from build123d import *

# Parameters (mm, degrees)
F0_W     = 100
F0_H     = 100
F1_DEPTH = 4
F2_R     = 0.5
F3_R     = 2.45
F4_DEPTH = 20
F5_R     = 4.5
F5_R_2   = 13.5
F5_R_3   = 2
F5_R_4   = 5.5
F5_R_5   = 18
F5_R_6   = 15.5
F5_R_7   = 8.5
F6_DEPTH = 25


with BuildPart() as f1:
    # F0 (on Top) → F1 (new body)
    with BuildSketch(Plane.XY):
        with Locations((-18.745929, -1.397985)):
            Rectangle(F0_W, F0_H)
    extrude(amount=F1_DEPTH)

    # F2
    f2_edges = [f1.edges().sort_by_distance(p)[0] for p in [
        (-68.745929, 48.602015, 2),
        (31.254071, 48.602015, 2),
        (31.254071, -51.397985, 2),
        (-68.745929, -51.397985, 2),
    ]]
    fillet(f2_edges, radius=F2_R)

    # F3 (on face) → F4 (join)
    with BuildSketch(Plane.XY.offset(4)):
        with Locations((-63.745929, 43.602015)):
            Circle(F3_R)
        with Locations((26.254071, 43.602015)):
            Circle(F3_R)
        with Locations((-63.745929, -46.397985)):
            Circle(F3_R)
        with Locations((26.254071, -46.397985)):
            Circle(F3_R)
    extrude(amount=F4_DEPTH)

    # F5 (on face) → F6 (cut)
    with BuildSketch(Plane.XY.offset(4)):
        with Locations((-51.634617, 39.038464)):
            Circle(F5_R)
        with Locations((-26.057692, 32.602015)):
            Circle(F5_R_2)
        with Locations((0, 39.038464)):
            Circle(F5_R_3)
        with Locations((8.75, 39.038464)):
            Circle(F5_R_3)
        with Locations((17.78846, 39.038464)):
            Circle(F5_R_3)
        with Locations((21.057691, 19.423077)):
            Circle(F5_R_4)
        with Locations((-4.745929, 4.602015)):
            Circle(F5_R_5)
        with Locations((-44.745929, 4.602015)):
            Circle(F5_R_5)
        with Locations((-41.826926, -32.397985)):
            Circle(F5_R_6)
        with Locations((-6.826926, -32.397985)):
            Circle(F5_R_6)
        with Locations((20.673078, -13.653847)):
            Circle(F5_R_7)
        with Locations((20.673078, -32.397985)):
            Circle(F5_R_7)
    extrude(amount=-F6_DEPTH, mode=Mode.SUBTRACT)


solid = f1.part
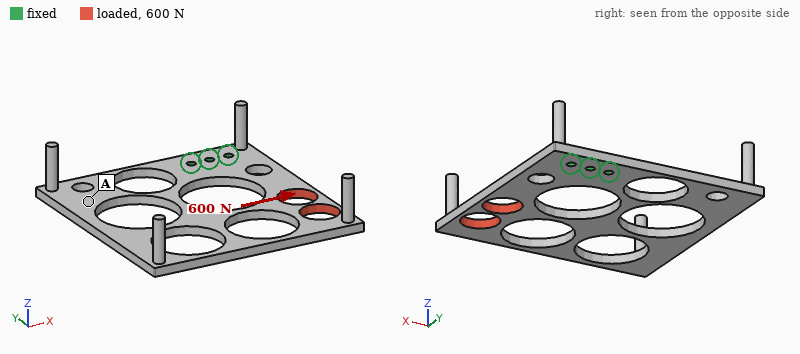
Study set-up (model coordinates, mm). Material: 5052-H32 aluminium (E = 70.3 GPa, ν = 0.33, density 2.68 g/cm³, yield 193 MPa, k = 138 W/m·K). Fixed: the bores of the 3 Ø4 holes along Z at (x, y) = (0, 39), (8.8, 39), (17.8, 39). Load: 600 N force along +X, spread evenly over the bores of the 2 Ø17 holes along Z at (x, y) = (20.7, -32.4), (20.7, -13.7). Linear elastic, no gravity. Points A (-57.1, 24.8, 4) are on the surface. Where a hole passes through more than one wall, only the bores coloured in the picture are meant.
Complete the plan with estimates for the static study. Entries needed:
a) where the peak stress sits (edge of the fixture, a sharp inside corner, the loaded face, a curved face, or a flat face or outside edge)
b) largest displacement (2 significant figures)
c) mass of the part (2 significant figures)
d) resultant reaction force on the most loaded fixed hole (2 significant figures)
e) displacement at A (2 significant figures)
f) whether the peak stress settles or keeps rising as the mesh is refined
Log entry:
edge of the fixture
0.25 mm
60 g
1.8 kN
0.13 mm
keeps rising
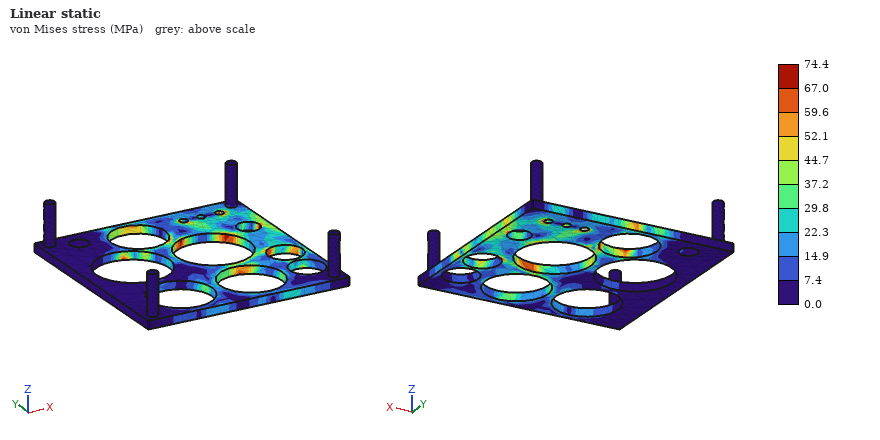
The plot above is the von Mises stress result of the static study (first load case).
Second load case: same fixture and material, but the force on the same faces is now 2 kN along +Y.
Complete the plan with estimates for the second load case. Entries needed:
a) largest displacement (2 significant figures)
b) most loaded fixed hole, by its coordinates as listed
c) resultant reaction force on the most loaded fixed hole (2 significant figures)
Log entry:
78 µm
(17.8, 39)
2.0 kN
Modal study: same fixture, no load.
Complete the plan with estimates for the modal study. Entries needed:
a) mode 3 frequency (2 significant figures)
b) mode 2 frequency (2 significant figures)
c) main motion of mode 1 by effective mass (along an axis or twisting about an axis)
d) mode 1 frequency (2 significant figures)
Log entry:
740 Hz
400 Hz
along Z
220 Hz
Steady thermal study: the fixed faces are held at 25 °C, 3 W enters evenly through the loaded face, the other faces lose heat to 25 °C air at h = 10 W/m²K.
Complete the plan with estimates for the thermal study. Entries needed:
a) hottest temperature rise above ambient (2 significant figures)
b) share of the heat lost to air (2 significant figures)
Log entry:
14 K
26 %
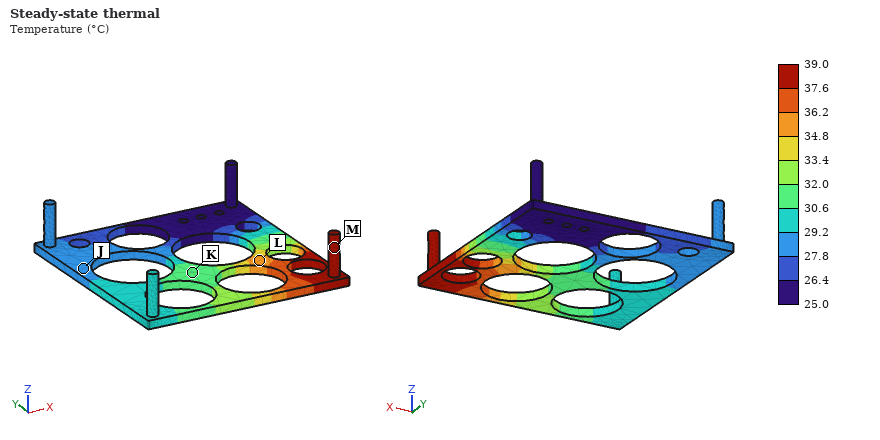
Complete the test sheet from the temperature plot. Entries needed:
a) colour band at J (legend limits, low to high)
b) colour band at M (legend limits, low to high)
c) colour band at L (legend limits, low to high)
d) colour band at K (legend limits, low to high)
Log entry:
27.8 to 29.2 °C
37.6 to 39.0 °C
34.8 to 36.2 °C
30.6 to 32.0 °C
